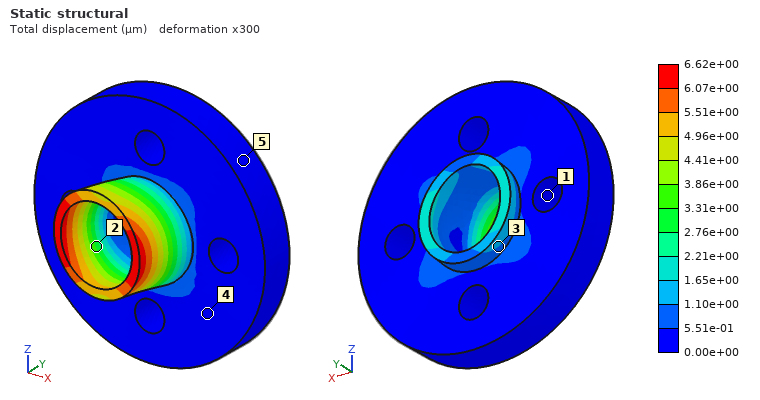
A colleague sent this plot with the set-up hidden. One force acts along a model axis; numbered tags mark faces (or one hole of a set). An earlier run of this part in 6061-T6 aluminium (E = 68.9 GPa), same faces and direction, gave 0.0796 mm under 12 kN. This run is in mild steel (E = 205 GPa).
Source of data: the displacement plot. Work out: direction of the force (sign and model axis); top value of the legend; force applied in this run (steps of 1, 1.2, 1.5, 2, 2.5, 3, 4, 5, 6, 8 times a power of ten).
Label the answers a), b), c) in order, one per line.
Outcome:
a) -X
b) 6.62e+00 µm
c) 3 kN
